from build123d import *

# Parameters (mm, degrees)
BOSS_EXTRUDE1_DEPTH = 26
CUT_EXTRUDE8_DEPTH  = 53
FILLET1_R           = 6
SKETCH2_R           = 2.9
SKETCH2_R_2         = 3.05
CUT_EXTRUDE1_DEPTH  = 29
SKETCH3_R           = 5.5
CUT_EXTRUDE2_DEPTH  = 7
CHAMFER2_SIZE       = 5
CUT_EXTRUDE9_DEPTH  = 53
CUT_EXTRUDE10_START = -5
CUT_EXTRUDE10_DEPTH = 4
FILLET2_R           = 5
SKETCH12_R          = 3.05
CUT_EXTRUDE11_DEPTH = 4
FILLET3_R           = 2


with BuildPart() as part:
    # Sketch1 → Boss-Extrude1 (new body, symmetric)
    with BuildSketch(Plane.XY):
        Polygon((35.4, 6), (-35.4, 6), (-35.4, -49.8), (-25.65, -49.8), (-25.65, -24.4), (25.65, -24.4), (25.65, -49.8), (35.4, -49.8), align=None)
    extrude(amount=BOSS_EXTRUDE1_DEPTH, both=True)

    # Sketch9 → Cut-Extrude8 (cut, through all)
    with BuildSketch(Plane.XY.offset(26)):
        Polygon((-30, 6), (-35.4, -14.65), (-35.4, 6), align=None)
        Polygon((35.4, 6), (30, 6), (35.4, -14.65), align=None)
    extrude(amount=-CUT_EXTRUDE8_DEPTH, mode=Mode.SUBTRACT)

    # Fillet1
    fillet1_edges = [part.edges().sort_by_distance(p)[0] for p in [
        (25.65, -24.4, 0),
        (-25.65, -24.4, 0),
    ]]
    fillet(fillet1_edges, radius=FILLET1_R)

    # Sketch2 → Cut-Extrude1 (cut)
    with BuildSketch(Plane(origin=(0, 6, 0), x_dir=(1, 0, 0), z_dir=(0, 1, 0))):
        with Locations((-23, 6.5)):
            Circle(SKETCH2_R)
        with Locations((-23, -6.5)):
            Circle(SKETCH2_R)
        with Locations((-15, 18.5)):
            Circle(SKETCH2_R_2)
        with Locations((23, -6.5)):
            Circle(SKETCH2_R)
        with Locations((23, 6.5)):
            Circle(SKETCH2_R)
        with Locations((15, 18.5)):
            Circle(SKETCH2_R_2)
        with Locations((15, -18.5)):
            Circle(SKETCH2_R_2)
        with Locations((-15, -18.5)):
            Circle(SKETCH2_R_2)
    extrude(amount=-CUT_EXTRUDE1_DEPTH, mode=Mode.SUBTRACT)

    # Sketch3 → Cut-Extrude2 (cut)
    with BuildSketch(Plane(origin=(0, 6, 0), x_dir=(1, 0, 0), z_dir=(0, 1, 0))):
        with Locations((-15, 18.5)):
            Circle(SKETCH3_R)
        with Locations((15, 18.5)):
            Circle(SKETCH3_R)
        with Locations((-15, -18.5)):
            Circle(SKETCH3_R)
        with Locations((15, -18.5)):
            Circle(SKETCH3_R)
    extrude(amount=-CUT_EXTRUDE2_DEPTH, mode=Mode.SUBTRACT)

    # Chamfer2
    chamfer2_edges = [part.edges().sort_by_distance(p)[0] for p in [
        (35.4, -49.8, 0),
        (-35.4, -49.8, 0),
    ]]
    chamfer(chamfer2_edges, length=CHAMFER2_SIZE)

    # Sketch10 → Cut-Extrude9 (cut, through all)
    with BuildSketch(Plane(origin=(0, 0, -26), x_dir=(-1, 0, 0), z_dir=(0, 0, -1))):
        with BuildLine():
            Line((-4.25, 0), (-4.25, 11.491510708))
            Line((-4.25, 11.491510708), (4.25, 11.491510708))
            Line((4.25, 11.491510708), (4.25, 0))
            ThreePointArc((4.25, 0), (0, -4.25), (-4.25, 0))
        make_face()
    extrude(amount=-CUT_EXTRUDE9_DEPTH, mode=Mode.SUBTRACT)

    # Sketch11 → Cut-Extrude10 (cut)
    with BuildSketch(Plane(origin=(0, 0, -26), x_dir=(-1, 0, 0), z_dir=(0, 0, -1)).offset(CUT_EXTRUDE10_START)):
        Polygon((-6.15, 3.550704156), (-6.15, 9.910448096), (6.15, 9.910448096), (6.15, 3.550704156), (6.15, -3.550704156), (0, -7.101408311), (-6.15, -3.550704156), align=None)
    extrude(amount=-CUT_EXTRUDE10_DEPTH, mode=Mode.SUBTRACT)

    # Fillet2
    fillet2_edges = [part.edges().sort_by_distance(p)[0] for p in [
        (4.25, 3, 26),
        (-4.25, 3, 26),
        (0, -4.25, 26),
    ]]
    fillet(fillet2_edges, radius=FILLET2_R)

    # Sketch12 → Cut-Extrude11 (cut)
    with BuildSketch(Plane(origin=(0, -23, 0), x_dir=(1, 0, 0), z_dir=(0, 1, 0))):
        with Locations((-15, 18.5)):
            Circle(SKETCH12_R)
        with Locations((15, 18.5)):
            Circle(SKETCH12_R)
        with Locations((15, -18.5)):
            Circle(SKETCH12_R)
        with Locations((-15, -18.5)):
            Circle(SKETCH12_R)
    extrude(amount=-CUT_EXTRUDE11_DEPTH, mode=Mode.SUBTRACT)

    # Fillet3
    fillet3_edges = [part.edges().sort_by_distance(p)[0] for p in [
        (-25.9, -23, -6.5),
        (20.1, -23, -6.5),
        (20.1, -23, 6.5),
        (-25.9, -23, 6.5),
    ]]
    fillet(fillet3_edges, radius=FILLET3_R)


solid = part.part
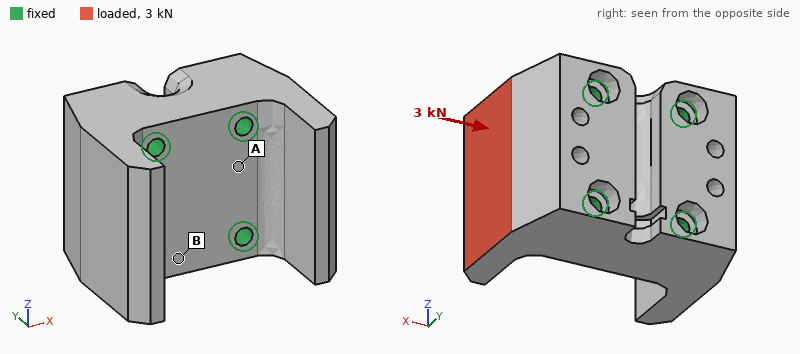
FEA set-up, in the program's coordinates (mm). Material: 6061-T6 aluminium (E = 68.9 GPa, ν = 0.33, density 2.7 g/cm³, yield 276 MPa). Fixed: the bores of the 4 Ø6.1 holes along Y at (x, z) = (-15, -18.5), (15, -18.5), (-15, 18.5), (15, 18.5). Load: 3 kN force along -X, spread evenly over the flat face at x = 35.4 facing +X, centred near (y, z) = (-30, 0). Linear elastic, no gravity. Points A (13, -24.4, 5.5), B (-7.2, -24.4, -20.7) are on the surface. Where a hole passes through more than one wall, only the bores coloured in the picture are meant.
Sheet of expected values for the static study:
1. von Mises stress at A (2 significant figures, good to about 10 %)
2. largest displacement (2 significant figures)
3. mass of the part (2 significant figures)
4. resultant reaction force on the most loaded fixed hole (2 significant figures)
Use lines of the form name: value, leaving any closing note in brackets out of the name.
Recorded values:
von Mises stress at A: 6.3 MPa
largest displacement: 24 µm
mass of the part: 320 g
resultant reaction force on the most loaded fixed hole: 1.3 kN
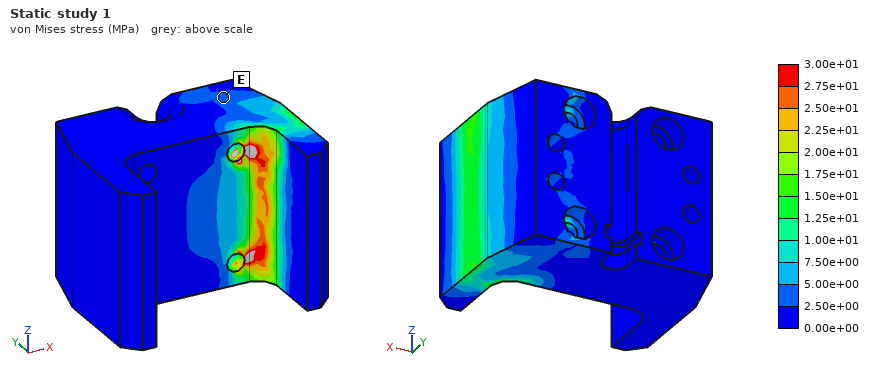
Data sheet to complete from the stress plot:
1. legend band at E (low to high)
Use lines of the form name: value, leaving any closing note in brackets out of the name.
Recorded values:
legend band at E: 2.50e+00 to 5.00e+00 MPa
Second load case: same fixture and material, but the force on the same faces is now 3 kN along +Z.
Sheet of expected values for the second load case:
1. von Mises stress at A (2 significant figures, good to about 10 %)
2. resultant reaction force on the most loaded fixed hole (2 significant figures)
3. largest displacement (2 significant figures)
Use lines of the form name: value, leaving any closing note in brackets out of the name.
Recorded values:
von Mises stress at A: 3.6 MPa
resultant reaction force on the most loaded fixed hole: 2.3 kN
largest displacement: 9.3 µm
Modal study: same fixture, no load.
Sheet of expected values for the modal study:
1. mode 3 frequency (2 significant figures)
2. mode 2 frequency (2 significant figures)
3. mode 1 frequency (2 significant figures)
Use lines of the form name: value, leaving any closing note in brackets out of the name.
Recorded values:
mode 3 frequency: 13 kHz
mode 2 frequency: 9100 Hz
mode 1 frequency: 9100 Hz
